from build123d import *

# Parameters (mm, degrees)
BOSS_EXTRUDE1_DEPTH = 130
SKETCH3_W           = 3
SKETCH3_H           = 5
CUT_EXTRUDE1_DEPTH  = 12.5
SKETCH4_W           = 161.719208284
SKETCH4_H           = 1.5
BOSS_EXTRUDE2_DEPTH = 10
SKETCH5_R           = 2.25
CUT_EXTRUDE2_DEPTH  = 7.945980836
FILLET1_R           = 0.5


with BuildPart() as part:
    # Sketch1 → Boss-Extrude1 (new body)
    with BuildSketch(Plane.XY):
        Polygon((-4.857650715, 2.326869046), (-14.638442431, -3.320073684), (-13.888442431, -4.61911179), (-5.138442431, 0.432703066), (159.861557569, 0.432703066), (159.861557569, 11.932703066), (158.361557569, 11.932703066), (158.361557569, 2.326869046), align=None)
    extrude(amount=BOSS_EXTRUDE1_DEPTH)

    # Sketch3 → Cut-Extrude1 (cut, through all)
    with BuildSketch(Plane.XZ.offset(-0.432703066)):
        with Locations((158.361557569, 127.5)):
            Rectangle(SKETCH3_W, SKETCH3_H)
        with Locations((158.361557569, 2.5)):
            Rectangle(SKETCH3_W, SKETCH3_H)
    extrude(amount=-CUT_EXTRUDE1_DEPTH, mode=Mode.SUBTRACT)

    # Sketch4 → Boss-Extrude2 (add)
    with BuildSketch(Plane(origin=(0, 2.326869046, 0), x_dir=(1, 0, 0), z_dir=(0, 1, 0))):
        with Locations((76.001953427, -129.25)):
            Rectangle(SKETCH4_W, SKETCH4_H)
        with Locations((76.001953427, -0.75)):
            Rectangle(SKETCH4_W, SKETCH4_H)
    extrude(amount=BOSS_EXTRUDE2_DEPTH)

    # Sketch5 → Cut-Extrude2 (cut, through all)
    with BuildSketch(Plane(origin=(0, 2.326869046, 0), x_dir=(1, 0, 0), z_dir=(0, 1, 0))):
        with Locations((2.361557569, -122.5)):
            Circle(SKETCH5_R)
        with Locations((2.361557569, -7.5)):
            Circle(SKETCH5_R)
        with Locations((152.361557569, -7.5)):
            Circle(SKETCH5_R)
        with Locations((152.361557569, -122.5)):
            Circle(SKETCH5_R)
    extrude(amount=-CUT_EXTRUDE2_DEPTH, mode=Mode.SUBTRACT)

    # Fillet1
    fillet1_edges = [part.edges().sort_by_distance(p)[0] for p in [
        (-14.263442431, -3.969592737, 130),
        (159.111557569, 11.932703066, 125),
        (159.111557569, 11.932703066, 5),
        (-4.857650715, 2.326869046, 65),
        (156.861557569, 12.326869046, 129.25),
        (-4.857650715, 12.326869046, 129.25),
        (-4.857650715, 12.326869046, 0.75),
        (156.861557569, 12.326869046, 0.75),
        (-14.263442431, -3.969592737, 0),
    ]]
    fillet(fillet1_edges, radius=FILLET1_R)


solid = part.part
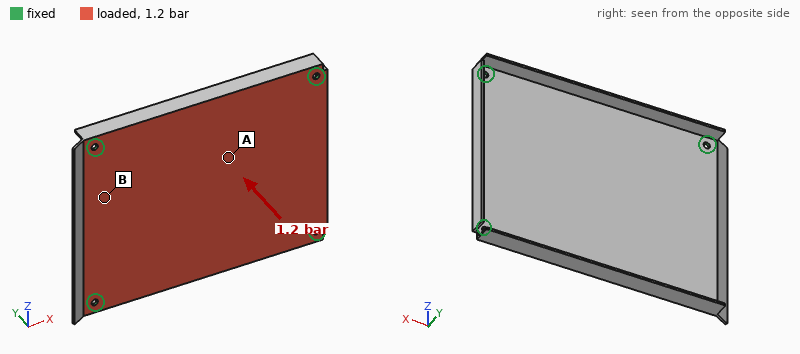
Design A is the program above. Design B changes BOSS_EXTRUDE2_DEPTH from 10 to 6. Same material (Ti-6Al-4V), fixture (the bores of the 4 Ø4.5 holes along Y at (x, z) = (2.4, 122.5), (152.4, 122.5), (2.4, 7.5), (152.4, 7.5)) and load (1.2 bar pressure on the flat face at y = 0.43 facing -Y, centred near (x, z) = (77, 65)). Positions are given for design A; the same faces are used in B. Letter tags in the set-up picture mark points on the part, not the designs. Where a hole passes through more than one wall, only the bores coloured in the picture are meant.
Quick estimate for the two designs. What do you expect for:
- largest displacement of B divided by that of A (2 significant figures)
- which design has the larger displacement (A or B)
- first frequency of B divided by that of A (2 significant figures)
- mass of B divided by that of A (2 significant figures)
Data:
1.1
B
0.95
0.96
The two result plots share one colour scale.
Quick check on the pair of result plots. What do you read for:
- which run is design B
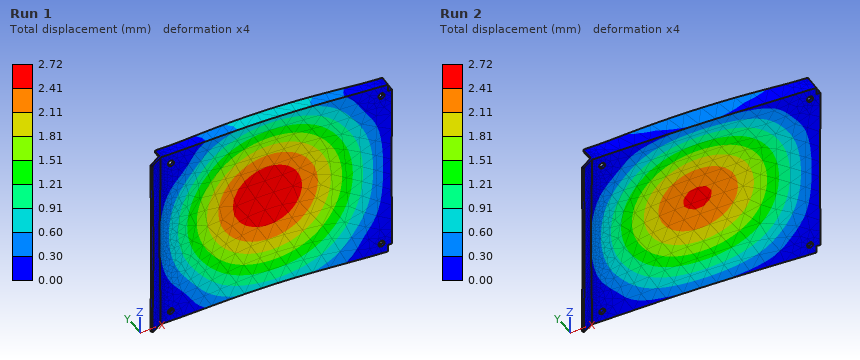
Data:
Run 1
